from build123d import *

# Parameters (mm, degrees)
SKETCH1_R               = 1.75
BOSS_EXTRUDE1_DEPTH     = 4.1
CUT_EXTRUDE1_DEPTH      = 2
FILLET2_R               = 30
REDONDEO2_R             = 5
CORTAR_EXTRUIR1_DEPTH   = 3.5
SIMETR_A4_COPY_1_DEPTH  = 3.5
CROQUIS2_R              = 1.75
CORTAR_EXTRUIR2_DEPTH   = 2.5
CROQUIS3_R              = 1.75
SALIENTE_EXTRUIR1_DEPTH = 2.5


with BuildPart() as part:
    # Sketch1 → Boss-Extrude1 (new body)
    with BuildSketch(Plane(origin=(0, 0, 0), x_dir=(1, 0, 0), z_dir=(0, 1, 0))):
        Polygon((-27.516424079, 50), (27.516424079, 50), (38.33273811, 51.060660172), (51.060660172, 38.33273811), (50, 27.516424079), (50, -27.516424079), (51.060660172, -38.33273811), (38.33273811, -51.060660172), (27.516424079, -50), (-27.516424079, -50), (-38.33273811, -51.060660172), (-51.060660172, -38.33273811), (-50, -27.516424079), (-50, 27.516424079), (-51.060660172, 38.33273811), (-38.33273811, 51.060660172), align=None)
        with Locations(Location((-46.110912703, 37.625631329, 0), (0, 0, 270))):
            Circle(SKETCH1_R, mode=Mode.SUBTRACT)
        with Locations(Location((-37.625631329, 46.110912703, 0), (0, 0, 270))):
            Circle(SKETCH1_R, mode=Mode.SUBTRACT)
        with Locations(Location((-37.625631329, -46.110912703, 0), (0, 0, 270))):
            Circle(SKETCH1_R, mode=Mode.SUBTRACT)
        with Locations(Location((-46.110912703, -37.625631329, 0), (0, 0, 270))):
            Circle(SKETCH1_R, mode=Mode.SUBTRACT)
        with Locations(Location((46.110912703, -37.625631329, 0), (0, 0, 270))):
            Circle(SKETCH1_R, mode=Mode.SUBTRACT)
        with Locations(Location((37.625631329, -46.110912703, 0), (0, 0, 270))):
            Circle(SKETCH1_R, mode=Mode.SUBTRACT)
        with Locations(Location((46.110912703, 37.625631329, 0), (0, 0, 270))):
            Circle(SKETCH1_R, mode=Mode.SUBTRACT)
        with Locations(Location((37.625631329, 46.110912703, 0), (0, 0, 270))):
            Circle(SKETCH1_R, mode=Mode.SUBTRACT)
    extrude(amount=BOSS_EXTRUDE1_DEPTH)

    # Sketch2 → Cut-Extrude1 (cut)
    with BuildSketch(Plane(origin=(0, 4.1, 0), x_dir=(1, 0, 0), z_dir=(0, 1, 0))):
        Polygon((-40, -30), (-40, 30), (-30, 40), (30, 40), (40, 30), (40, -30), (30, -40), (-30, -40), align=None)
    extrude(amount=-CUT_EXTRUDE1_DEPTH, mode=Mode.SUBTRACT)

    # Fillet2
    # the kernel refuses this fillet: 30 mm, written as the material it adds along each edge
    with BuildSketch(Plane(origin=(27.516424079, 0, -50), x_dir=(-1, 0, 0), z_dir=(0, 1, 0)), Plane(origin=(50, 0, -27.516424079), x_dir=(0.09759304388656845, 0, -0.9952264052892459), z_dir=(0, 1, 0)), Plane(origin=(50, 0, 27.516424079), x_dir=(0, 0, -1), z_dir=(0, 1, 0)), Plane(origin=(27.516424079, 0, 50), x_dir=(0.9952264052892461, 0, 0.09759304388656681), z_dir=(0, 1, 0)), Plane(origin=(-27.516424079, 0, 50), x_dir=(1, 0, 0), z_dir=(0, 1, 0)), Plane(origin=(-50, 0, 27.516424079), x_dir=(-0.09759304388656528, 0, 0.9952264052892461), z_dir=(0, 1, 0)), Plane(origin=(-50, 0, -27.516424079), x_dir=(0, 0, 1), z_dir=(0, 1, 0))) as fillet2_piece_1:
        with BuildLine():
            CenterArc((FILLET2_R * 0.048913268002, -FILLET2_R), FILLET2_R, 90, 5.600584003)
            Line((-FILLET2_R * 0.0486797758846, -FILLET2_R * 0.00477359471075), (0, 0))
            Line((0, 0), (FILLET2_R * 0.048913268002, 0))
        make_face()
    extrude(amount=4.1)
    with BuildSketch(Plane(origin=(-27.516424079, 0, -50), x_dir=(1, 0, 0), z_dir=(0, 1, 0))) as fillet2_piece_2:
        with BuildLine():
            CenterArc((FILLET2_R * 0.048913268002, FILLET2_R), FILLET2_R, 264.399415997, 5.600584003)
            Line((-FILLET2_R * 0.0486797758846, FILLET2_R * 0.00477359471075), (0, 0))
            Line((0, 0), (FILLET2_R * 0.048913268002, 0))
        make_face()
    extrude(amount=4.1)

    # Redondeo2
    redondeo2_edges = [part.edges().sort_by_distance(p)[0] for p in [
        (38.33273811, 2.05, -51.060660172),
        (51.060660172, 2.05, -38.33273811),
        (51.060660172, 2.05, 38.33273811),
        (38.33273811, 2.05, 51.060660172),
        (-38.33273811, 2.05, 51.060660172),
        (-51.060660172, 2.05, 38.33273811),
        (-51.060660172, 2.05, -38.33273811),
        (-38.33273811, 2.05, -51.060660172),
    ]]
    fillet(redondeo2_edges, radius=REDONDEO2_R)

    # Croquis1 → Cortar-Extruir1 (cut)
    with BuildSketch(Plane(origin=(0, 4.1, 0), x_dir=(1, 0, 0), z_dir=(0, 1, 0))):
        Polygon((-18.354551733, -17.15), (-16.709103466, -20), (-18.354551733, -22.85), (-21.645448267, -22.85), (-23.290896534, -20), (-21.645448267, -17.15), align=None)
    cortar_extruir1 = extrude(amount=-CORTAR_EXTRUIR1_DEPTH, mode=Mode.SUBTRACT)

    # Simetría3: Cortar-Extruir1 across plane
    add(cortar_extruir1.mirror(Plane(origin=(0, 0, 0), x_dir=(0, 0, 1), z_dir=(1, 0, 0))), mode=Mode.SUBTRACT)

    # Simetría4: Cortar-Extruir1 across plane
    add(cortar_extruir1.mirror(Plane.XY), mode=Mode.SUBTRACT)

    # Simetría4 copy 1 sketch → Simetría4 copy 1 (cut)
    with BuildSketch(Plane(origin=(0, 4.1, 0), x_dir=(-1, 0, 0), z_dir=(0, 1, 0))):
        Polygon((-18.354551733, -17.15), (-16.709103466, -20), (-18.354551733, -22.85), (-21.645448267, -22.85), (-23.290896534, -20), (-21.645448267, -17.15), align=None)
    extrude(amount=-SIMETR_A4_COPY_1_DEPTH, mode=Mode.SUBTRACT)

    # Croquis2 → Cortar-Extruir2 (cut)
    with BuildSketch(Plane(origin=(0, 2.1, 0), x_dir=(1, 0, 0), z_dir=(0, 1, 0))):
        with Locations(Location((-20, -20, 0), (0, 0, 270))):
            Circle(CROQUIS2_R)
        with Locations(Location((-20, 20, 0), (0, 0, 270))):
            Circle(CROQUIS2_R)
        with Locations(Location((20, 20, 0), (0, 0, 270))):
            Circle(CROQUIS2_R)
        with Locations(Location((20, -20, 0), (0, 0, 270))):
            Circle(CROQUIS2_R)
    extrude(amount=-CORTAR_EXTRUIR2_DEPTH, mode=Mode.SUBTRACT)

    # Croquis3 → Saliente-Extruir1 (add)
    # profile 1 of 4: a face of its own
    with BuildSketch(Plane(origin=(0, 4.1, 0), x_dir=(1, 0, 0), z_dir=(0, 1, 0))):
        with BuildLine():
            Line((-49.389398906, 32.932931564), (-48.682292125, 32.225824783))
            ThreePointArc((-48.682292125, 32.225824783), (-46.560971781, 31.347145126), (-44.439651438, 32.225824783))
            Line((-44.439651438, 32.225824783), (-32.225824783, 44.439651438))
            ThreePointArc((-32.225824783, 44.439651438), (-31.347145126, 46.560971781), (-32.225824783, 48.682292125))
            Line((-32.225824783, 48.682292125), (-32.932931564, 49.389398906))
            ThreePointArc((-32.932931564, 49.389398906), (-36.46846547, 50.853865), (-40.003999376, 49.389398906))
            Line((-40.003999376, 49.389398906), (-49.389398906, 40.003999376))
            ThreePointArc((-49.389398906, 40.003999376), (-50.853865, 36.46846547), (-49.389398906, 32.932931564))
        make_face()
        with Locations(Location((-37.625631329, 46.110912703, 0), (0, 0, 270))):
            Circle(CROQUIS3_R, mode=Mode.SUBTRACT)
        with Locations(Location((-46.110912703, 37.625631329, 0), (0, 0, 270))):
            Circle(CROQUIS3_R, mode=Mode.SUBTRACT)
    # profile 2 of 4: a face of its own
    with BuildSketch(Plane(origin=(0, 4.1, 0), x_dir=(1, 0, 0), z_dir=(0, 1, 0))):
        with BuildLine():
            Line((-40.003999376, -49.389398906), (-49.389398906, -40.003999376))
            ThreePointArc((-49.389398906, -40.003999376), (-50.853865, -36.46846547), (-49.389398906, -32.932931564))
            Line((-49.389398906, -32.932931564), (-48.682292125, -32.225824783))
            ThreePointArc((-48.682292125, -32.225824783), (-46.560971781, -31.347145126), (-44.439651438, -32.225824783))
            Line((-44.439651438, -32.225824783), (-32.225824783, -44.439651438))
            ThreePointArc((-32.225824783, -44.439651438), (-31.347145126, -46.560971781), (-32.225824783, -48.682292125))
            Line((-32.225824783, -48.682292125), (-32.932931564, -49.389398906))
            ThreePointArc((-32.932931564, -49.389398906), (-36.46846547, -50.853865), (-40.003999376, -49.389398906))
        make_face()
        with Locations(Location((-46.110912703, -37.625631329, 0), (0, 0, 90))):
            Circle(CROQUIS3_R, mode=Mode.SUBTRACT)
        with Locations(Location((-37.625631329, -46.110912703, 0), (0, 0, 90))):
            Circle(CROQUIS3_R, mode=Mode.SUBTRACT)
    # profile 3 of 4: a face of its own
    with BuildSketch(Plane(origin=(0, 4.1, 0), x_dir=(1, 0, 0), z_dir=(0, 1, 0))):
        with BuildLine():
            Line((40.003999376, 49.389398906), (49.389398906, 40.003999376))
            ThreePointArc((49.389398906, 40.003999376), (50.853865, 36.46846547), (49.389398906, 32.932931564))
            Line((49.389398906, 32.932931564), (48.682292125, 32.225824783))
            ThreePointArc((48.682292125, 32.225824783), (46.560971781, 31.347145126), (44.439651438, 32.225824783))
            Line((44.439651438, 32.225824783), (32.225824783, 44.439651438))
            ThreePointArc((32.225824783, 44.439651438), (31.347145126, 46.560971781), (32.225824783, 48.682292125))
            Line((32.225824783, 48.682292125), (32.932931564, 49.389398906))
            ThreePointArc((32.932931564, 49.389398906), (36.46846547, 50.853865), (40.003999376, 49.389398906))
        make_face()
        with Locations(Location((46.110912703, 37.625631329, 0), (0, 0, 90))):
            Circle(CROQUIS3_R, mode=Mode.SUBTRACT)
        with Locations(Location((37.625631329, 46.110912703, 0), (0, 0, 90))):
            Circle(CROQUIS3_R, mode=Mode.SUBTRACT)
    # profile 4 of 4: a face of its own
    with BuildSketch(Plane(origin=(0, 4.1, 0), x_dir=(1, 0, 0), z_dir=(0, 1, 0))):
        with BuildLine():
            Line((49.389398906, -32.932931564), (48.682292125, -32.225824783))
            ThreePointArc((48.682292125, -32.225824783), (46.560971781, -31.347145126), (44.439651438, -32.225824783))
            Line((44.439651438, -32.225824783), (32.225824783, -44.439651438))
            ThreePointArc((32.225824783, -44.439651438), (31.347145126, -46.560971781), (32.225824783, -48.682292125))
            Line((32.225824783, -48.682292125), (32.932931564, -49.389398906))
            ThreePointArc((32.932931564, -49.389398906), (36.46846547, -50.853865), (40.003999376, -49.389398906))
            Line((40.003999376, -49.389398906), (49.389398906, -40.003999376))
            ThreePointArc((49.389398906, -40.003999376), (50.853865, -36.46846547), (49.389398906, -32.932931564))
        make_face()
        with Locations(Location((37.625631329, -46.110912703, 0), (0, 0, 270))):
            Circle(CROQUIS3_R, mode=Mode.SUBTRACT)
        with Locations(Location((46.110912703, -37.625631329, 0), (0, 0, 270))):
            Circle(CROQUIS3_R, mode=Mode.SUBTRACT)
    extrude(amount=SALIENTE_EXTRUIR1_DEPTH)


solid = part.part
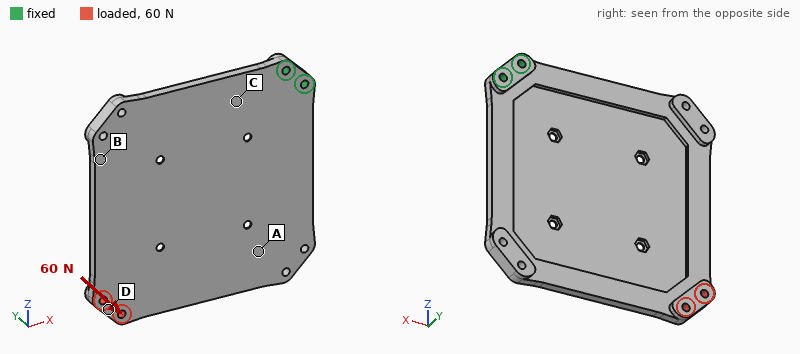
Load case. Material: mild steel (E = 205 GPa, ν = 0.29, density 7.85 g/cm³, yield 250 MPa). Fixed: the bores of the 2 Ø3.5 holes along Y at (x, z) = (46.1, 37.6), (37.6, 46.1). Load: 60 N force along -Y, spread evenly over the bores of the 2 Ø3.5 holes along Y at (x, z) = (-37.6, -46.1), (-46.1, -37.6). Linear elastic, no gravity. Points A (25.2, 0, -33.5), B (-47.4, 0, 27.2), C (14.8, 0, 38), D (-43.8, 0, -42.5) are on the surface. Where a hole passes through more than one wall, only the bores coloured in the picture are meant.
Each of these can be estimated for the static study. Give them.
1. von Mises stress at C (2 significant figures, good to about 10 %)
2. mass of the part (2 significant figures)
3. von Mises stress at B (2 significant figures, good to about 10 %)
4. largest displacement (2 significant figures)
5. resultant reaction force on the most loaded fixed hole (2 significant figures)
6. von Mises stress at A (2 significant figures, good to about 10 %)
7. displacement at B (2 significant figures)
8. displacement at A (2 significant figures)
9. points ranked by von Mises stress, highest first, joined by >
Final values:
49 MPa
230 g
24 MPa
1.0 mm
260 N
14 MPa
0.44 mm
0.36 mm
C > B > A > D
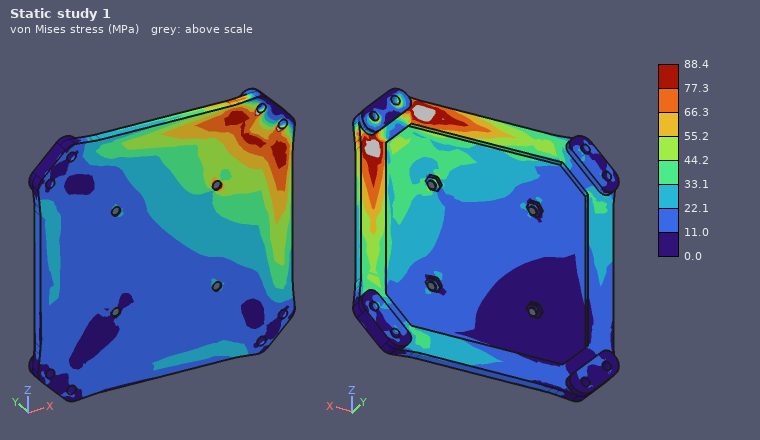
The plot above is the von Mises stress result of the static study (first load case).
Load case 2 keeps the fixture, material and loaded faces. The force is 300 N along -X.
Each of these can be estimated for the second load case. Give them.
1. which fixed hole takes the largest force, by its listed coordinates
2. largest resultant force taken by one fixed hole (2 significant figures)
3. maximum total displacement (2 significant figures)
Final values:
(46.1, 37.6)
1.7 kN
0.12 mm
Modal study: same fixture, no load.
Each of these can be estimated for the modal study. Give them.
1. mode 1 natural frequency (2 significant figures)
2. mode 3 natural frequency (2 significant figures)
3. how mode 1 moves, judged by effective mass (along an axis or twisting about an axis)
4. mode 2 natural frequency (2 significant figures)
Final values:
170 Hz
770 Hz
along Y
360 Hz
